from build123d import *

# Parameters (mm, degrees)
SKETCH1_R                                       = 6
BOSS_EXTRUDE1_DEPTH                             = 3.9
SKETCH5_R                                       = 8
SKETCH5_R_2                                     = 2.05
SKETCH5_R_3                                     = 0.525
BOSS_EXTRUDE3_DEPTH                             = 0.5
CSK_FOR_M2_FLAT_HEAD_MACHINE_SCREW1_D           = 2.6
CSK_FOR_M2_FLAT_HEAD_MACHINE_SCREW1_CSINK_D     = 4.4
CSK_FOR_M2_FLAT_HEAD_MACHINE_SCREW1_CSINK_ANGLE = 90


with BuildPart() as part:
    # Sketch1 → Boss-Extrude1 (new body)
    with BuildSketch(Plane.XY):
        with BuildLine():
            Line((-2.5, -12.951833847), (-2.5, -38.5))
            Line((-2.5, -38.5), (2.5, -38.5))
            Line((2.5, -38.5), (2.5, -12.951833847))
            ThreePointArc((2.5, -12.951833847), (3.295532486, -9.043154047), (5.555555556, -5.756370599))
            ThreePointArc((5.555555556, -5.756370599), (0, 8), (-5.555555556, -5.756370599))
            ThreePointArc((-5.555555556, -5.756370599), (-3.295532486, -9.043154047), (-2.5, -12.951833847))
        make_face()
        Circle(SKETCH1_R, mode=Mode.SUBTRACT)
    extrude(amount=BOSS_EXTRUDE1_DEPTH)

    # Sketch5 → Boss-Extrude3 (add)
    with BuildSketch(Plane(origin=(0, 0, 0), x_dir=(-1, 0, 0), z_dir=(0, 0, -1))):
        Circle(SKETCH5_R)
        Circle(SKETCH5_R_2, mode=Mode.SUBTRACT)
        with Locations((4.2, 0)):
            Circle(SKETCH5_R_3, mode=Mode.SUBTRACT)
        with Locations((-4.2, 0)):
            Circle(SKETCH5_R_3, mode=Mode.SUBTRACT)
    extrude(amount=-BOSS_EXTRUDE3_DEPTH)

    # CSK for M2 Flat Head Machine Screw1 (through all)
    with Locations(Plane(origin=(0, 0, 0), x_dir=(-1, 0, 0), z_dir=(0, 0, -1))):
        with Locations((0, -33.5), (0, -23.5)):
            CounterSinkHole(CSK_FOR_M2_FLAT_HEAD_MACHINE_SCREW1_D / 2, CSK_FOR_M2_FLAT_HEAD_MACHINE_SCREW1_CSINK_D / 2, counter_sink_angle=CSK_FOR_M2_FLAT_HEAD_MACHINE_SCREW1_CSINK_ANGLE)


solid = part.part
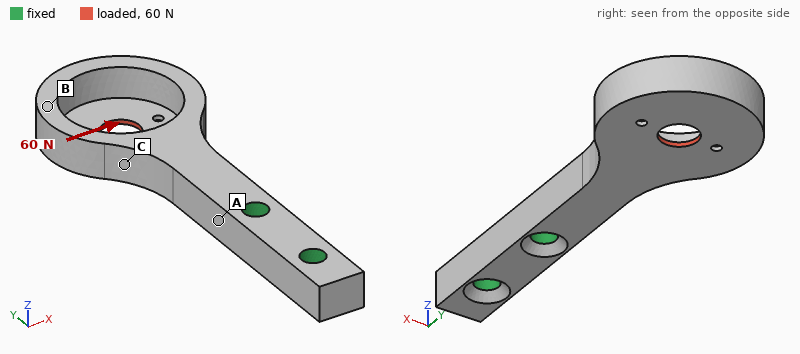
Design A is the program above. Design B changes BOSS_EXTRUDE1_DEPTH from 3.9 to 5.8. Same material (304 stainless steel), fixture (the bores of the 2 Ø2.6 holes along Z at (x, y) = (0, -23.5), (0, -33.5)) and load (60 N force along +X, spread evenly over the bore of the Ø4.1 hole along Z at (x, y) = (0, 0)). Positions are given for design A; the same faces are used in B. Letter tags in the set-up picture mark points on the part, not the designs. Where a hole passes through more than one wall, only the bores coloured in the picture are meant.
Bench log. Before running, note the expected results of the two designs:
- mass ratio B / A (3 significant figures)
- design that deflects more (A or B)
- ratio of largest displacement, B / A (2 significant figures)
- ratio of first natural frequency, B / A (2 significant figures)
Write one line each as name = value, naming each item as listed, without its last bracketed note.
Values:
mass ratio B / A = 1.47
design that deflects more = A
ratio of largest displacement, B / A = 0.68
ratio of first natural frequency, B / A = 1.3
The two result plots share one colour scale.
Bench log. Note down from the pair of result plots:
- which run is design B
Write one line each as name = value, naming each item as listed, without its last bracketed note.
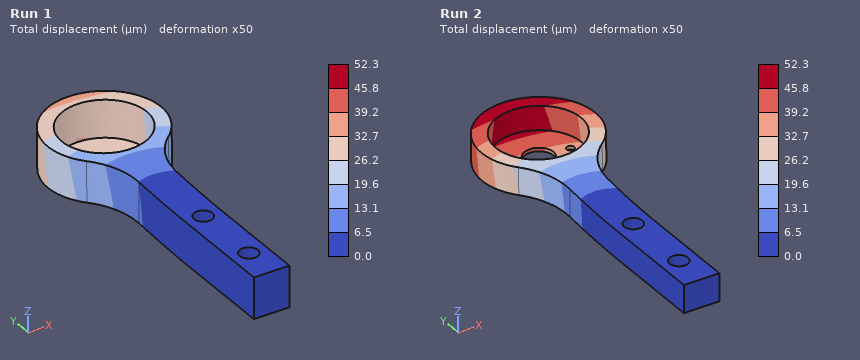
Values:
which run is design B = Run 1
